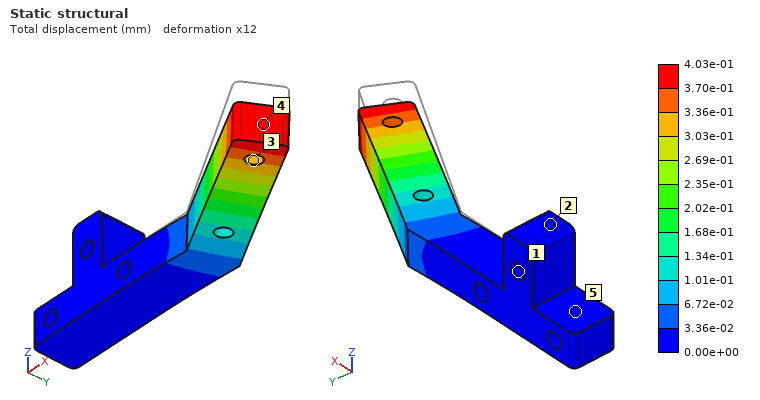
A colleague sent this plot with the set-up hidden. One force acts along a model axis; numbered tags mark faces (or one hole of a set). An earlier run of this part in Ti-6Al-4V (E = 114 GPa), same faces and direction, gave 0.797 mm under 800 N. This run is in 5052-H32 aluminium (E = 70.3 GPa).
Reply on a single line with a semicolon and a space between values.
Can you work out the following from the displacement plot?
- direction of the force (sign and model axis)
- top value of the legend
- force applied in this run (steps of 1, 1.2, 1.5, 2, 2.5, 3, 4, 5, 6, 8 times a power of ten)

-Z; 4.03e-01 mm; 250 N
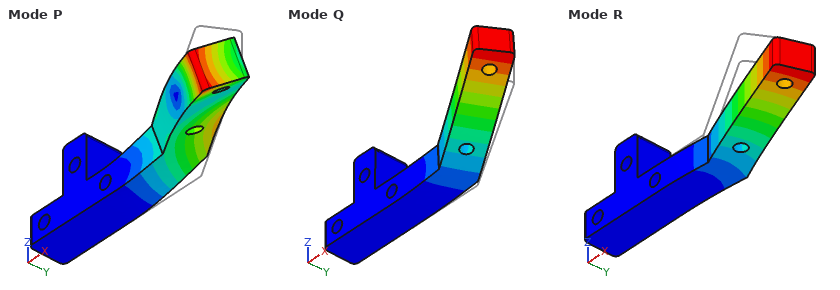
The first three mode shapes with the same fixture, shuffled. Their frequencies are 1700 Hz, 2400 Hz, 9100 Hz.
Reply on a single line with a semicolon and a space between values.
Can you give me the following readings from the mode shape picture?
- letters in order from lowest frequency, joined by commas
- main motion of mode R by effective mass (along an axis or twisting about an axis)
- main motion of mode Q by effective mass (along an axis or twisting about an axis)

Q, R, P; along Y; along Z
